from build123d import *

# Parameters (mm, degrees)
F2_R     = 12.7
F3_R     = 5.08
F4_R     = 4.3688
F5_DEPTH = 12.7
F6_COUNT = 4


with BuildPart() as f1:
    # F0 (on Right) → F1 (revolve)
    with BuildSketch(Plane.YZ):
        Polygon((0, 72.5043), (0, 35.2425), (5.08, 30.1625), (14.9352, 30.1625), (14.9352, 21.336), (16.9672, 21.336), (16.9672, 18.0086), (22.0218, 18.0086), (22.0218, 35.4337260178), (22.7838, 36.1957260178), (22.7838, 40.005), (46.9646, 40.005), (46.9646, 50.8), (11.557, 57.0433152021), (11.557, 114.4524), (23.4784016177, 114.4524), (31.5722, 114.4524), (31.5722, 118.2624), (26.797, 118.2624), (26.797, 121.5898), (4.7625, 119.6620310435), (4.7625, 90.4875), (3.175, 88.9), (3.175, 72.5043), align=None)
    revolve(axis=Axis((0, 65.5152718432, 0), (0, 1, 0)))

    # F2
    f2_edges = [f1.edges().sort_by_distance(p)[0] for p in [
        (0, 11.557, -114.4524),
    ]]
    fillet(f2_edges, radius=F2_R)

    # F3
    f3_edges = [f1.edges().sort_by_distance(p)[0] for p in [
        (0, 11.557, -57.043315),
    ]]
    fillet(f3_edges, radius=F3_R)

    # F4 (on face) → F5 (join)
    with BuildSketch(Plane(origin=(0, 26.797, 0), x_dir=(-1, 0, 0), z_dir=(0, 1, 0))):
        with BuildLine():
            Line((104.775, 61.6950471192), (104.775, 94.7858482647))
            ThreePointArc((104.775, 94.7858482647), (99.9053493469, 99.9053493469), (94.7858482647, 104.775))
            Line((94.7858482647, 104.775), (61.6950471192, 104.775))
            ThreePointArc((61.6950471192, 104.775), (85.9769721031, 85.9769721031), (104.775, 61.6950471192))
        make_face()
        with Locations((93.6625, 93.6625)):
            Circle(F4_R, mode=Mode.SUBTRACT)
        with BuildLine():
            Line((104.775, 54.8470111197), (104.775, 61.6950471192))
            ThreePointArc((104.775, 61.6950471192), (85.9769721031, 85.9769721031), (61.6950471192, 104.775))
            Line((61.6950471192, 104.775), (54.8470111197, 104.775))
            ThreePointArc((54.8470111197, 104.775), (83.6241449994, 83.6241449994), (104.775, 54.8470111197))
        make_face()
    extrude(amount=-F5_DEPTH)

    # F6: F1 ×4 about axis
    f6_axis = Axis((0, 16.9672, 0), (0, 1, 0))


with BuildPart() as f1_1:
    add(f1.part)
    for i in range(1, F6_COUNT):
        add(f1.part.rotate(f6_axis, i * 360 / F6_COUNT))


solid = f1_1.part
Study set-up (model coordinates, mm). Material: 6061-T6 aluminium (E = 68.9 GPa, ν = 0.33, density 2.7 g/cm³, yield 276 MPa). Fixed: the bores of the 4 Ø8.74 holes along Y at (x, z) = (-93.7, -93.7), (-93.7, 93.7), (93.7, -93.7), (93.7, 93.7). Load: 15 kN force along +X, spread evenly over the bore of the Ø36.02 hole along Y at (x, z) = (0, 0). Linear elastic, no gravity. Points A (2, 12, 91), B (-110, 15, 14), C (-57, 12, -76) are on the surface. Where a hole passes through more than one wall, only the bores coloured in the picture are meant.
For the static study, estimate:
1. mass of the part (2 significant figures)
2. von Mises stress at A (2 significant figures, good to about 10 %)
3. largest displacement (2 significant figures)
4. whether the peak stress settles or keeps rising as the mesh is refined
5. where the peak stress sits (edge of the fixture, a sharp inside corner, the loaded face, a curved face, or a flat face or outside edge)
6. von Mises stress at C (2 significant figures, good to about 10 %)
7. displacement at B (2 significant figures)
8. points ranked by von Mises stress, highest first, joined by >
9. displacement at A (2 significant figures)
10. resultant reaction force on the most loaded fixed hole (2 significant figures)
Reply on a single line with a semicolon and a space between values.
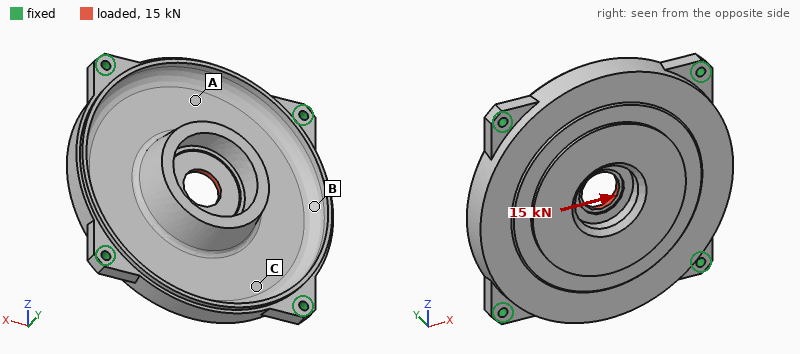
1.9 kg; 11 MPa; 69 µm; keeps rising; edge of the fixture; 18 MPa; 26 µm; C > A > B; 16 µm; 3.8 kN
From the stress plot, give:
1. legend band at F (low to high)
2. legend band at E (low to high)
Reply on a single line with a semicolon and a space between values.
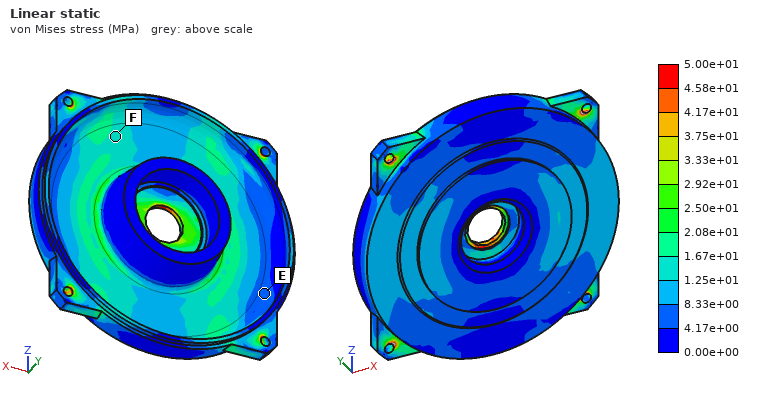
1.25e+01 to 1.67e+01 MPa; 4.17e+00 to 8.33e+00 MPa
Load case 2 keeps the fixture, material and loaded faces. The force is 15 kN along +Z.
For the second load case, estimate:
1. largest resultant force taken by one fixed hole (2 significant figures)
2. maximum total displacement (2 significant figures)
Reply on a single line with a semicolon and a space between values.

3.8 kN; 69 µm
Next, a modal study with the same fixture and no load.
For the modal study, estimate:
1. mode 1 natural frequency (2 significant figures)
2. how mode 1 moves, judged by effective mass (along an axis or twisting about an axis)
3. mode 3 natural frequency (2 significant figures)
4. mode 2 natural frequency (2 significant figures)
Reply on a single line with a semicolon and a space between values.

1300 Hz; along Y; 2000 Hz; 2000 Hz
